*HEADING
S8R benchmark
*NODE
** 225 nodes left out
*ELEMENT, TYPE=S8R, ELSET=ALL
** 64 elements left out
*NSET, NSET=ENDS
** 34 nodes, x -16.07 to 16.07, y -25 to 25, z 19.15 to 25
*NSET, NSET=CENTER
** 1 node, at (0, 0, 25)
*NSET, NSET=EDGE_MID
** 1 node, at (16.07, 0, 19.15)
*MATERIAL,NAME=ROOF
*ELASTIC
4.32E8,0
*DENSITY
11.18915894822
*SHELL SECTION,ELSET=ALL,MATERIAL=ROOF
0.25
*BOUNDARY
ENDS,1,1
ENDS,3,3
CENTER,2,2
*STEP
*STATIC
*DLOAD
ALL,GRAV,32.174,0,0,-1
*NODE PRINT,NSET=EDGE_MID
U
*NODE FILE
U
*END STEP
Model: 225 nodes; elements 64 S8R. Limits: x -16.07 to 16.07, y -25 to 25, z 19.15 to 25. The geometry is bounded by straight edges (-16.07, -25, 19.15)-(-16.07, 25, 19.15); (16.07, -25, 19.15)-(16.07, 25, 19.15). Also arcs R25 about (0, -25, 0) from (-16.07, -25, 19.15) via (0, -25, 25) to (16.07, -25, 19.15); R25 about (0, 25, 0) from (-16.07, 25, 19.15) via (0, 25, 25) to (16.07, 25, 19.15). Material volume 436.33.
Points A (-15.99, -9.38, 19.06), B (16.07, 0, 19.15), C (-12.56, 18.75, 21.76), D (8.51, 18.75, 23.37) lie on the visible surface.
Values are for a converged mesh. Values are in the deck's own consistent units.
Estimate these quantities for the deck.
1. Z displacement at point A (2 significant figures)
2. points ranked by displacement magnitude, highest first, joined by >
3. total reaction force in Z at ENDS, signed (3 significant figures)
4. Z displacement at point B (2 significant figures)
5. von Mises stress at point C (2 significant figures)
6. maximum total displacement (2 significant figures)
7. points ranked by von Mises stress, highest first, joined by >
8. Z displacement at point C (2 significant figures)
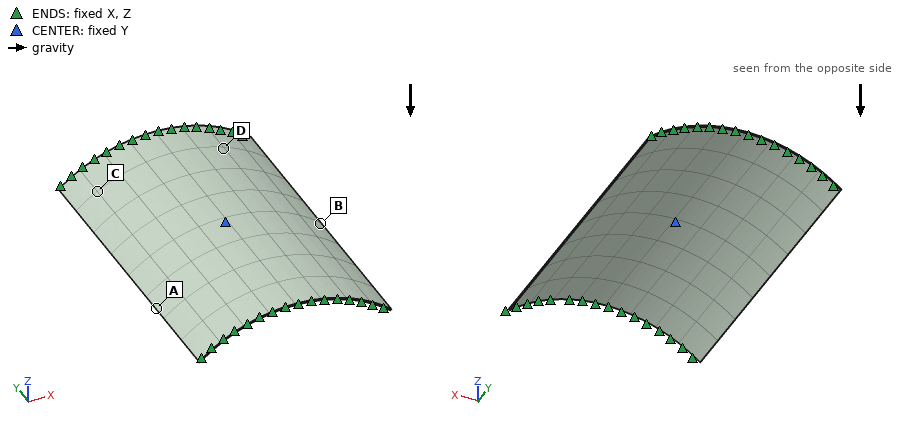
-0.25
B > A > C > D
1.57e+05
-0.30
2.4e+05
0.34
A > B > C > D
-0.079
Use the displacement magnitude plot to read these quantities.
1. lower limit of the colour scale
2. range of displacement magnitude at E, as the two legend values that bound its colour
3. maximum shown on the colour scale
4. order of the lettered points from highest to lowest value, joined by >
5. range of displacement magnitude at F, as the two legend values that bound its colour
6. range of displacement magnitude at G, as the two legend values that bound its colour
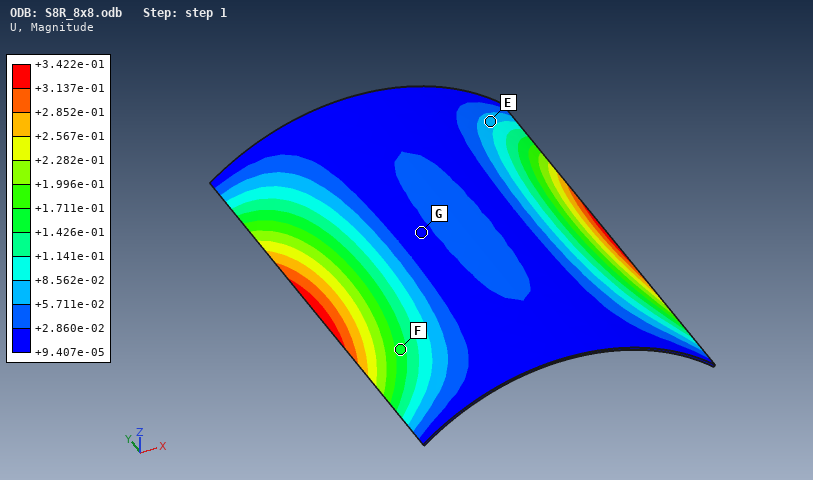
+9.407e-05
+5.711e-02 to +8.562e-02
+3.422e-01
F > E > G
+1.426e-01 to +1.711e-01
+9.407e-05 to +2.860e-02
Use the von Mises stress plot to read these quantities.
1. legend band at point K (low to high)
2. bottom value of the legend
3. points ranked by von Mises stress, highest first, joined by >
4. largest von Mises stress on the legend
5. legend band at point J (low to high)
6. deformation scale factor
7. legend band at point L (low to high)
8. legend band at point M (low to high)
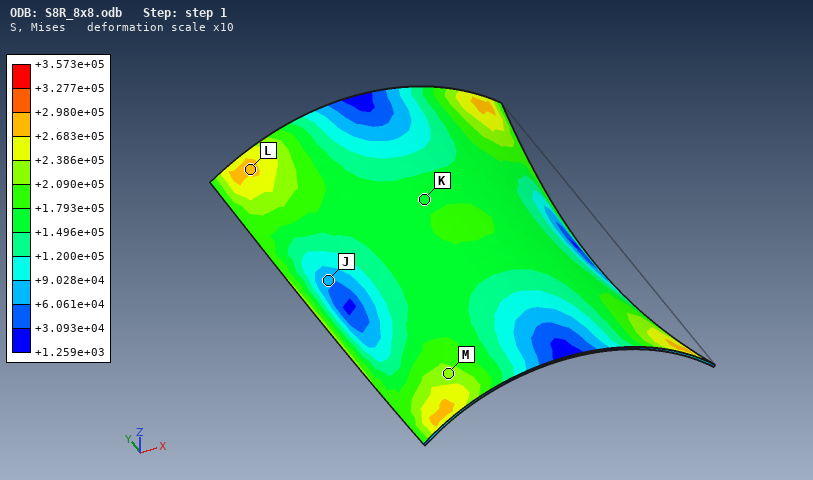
+1.496e+05 to +1.793e+05
+1.259e+03
L > M > K > J
+3.573e+05
+6.061e+04 to +9.028e+04
10
+2.683e+05 to +2.980e+05
+2.090e+05 to +2.386e+05
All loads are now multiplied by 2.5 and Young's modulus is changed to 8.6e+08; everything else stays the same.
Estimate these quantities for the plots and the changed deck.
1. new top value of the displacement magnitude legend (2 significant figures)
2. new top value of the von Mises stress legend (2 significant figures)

0.43
8.9e+05
